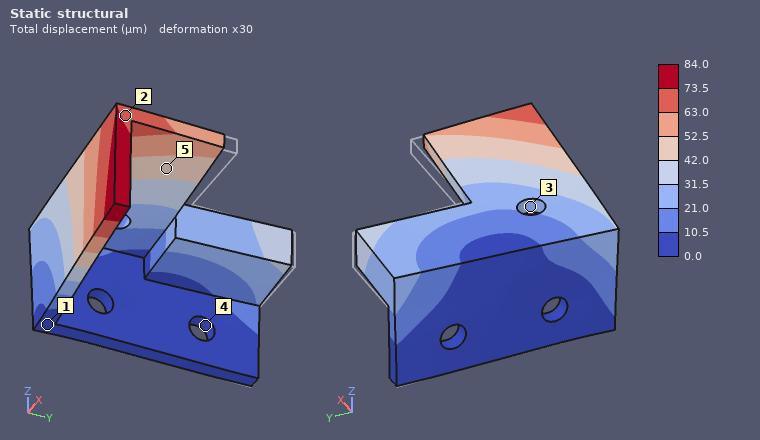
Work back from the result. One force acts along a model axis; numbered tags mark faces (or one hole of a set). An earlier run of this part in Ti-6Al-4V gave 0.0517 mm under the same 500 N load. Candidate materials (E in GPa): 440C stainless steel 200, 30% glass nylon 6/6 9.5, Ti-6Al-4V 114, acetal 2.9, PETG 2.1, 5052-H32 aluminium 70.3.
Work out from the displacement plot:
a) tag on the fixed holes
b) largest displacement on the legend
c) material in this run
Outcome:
4
84.0 µm
5052-H32 aluminium
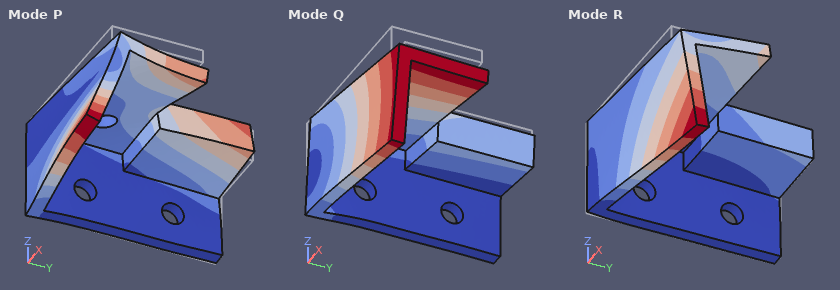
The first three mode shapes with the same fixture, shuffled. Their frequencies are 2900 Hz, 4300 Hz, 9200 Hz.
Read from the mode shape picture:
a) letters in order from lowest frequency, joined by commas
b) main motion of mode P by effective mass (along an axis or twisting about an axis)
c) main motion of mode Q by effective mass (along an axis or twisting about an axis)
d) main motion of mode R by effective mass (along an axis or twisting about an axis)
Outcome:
Q, R, P
along X
along Z
along Y
